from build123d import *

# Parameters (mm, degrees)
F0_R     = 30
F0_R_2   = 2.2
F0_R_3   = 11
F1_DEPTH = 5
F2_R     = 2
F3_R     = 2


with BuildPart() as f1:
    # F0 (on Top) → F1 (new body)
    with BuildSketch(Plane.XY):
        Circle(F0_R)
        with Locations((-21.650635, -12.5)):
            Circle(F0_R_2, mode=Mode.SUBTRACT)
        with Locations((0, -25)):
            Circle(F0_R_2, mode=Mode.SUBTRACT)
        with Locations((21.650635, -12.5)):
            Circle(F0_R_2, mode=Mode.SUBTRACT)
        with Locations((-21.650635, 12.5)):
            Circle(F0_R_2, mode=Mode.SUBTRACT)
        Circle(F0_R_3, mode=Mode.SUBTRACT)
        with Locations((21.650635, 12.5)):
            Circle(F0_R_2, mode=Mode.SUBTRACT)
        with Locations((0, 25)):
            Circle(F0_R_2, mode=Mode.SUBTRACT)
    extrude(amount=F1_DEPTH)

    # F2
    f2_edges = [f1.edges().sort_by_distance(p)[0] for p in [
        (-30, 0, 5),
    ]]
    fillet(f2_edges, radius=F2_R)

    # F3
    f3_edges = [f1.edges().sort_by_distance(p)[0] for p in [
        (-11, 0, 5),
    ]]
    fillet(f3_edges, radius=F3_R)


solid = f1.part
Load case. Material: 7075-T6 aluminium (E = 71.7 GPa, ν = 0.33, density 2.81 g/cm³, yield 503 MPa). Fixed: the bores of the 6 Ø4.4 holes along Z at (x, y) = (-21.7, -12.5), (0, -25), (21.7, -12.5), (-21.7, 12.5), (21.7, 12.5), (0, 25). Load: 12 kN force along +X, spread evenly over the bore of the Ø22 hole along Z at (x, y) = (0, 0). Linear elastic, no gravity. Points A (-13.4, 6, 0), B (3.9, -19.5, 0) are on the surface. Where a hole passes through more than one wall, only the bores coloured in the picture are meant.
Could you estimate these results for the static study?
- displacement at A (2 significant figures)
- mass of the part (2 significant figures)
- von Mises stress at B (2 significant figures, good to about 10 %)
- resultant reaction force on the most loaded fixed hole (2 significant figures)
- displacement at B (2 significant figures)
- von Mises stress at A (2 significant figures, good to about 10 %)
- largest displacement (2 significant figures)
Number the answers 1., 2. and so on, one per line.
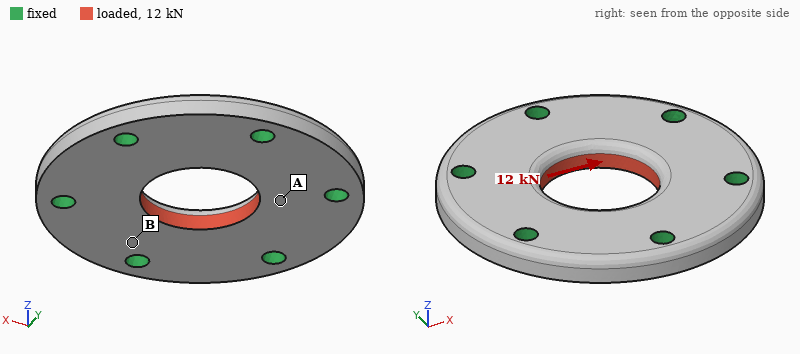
1. 8.2 µm
2. 32 g
3. 13 MPa
4. 2.6 kN
5. 2.8 µm
6. 59 MPa
7. 14 µm
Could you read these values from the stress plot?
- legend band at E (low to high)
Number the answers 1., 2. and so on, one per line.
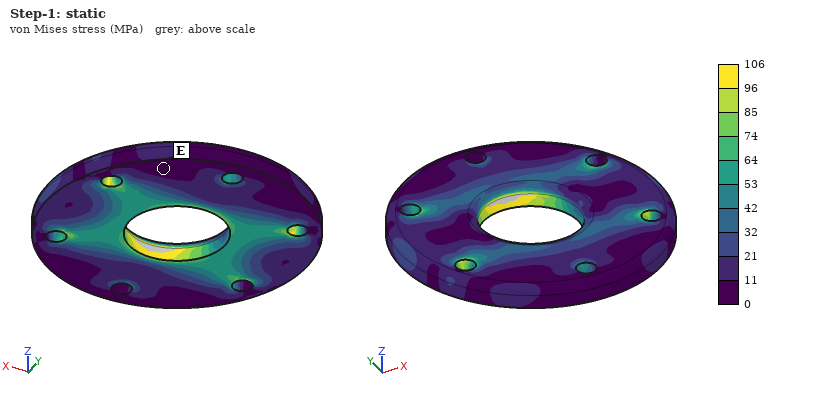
1. 0 to 11 MPa
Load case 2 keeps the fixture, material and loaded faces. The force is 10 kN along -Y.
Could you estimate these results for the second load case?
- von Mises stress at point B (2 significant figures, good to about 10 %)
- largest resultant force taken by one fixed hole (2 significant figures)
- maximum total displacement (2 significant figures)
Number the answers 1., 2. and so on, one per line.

1. 39 MPa
2. 2.4 kN
3. 11 µm
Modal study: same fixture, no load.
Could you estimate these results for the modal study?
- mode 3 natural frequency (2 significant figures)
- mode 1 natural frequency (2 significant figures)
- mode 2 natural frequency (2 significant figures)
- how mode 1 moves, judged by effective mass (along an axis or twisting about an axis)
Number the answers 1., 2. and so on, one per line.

1. 29 kHz
2. 22 kHz
3. 29 kHz
4. along Z
